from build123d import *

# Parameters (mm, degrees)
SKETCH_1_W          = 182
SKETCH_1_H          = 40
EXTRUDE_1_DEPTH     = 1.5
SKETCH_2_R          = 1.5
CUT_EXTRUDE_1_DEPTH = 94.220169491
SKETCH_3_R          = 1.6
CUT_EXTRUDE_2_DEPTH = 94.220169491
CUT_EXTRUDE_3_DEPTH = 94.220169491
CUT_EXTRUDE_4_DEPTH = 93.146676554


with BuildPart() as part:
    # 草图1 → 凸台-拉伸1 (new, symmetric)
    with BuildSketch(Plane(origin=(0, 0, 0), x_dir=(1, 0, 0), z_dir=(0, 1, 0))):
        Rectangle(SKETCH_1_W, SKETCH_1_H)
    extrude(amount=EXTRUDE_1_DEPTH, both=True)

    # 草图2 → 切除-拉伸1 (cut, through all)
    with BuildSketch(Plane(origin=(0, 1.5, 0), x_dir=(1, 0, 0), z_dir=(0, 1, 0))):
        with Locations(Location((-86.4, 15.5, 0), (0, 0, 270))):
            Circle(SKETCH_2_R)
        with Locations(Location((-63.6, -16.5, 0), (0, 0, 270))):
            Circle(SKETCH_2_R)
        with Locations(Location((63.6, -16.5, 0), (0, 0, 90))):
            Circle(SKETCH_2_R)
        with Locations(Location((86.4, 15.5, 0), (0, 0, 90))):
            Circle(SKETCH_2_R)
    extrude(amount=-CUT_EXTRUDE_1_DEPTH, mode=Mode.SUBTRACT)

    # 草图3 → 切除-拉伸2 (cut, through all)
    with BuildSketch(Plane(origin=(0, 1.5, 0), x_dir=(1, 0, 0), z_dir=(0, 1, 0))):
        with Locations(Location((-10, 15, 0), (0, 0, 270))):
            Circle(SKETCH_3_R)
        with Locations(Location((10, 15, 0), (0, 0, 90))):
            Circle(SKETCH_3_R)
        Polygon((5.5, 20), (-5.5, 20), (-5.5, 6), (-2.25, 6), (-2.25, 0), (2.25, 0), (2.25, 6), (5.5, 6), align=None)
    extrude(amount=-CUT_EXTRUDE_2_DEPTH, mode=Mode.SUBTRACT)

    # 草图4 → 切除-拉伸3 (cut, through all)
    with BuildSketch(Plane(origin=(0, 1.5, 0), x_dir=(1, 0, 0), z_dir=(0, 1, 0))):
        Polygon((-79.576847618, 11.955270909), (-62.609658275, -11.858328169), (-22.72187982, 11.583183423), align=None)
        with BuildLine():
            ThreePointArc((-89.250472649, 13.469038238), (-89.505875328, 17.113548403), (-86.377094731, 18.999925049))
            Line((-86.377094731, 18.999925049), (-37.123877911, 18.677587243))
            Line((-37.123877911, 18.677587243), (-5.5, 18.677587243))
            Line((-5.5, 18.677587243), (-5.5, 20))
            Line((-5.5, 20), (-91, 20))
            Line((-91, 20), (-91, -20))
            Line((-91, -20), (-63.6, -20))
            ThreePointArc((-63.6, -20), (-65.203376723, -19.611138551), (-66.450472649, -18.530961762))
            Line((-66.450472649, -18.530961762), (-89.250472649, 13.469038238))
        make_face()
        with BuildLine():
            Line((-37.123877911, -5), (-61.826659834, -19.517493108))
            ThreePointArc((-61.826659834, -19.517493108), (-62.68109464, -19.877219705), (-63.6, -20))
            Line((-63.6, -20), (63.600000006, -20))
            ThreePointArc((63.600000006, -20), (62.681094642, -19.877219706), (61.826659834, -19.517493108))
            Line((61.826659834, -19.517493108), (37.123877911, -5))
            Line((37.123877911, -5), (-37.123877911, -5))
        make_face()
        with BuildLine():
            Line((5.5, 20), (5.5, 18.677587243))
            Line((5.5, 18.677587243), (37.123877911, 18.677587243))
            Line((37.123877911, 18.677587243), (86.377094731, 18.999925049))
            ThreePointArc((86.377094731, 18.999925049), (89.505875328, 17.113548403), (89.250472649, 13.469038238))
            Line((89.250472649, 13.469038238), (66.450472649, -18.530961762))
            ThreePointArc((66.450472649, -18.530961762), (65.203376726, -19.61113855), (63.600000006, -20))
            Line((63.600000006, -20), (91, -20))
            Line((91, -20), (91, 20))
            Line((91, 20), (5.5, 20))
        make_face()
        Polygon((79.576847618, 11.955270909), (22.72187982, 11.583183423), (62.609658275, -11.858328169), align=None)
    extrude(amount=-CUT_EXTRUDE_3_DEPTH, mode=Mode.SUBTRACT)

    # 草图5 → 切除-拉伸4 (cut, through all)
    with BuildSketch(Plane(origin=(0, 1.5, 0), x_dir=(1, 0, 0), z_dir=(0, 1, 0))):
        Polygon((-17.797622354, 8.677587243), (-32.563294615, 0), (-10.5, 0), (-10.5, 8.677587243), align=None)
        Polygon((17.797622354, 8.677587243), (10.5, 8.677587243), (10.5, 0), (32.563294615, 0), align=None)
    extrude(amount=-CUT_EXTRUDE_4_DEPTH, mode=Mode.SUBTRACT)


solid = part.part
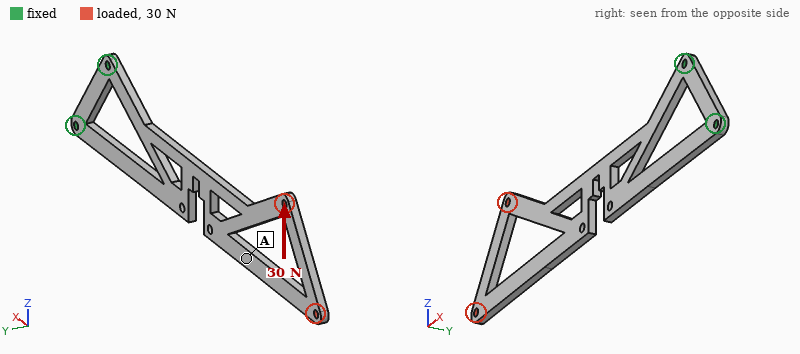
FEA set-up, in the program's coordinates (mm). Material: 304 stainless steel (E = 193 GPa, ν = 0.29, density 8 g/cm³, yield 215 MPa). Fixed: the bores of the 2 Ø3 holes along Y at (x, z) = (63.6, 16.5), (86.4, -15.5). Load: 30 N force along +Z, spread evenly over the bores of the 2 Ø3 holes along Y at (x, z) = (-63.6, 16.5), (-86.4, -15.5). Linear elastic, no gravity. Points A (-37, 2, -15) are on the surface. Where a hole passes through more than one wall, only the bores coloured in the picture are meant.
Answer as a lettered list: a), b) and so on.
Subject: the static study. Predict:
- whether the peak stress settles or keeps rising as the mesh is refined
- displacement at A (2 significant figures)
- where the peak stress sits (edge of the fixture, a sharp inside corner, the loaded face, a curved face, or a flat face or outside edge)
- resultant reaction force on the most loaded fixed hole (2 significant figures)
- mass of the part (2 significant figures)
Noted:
a) keeps rising
b) 0.21 mm
c) a sharp inside corner
d) 140 N
e) 68 g
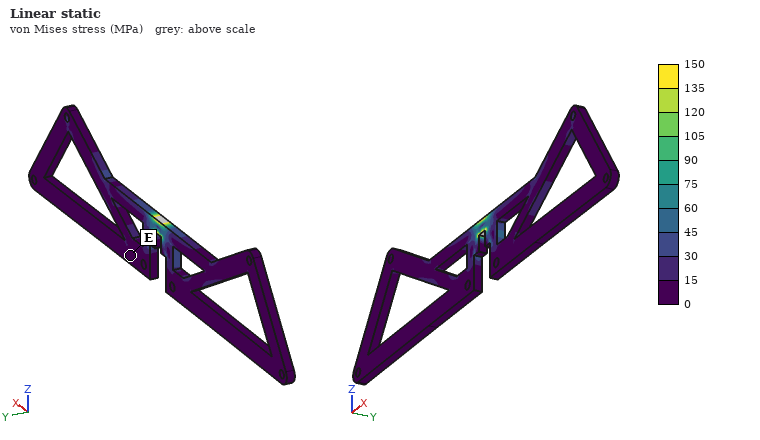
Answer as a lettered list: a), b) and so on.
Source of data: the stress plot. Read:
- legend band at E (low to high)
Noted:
a) 0 to 15 MPa
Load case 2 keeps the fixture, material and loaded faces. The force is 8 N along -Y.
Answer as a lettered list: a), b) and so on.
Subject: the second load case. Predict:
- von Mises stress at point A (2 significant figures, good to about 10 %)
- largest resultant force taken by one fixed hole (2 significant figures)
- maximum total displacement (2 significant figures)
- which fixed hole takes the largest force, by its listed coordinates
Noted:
a) 13 MPa
b) 13 N
c) 1.8 mm
d) (63.6, 16.5)
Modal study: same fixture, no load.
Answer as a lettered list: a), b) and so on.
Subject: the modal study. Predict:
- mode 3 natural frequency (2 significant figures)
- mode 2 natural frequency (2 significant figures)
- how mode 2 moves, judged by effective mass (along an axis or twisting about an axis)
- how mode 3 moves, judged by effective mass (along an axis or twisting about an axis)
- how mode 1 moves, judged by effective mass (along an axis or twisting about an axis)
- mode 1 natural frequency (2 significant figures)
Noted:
a) 470 Hz
b) 340 Hz
c) along Z
d) along Y
e) along Y
f) 84 Hz
